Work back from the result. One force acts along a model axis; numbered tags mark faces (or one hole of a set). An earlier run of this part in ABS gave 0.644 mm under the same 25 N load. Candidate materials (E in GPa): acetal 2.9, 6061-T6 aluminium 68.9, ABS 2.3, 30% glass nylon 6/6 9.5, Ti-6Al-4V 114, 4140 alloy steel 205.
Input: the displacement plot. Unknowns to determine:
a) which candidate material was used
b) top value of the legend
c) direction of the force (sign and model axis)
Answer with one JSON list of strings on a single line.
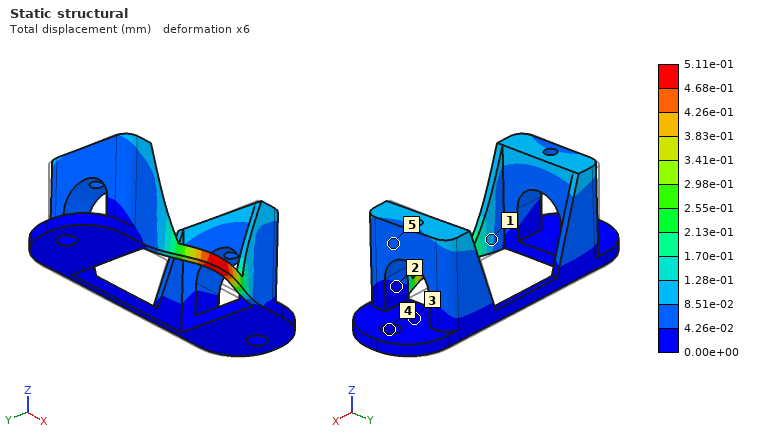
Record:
["acetal", "5.11e-01 mm", "-Y"]
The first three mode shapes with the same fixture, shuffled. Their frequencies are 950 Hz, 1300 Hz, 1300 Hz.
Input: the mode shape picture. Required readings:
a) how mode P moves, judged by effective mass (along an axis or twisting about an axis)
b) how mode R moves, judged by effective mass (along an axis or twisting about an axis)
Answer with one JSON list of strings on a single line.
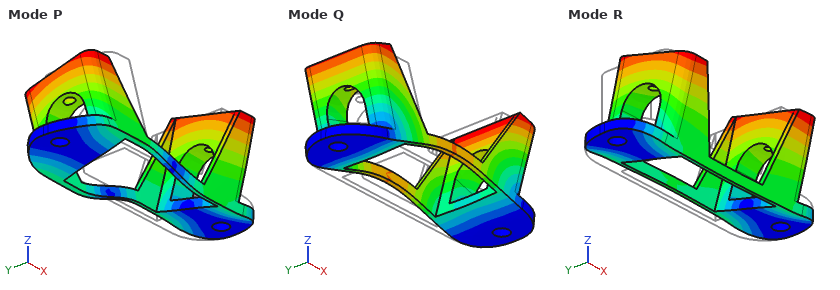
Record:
["twisting about Z", "along Y"]
